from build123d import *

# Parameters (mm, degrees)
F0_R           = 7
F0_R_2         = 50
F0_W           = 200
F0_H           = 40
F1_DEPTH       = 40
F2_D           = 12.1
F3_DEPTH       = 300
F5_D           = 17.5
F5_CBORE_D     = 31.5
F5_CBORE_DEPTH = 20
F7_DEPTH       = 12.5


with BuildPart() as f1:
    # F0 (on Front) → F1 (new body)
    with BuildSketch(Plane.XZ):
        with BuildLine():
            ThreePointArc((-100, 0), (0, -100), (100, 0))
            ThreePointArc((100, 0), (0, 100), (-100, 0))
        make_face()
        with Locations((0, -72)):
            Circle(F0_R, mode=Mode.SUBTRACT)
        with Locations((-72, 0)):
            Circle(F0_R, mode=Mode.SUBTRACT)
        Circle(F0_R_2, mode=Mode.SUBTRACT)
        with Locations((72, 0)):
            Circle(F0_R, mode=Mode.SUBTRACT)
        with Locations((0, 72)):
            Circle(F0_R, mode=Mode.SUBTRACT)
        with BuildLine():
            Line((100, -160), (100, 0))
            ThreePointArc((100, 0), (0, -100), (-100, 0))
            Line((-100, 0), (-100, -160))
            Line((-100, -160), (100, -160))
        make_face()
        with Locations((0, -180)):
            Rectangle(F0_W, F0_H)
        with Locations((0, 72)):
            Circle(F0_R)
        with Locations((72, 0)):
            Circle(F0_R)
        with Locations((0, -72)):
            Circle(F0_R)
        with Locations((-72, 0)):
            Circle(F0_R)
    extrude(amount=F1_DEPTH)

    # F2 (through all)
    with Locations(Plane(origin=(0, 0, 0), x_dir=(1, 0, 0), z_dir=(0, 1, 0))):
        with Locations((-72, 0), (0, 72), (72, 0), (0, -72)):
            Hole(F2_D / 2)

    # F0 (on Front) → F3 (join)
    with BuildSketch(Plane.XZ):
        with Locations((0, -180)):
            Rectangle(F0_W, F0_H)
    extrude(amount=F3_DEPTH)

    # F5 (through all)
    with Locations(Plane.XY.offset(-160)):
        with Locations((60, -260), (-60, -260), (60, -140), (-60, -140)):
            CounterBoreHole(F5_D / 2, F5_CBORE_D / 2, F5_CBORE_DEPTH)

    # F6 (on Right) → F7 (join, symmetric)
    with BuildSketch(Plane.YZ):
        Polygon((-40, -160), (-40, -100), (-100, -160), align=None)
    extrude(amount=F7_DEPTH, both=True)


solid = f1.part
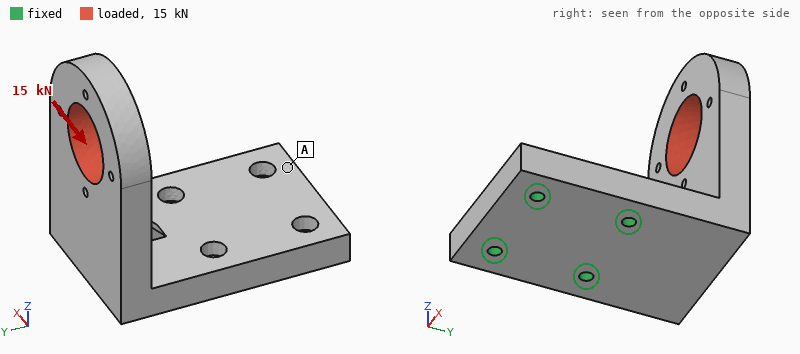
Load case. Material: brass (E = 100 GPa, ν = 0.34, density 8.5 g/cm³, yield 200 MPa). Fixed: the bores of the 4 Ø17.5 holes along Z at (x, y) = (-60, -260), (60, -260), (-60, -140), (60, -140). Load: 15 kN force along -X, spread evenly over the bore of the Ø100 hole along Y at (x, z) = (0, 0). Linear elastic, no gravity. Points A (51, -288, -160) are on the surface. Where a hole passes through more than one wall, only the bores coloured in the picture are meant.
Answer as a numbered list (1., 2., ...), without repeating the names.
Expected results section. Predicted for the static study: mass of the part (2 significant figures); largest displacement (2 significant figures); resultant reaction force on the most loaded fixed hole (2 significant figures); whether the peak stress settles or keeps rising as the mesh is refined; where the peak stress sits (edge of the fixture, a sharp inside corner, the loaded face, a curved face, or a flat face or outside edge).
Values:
1. 33 kg
2. 0.41 mm
3. 29 kN
4. keeps rising
5. edge of the fixture
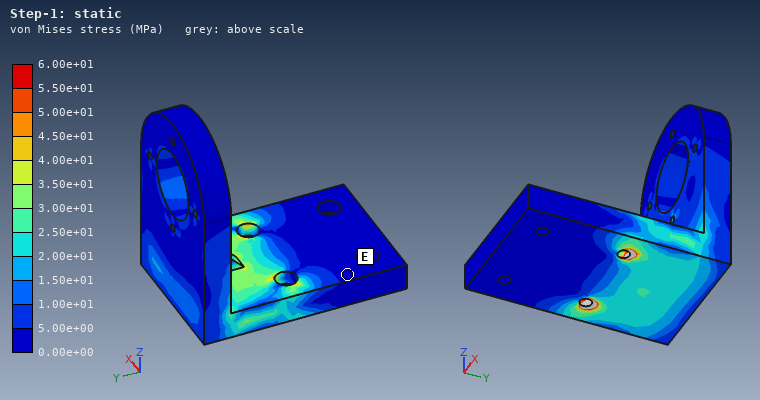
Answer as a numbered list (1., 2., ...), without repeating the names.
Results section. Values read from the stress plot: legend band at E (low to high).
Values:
1. 0.00e+00 to 5.00e+00 MPa
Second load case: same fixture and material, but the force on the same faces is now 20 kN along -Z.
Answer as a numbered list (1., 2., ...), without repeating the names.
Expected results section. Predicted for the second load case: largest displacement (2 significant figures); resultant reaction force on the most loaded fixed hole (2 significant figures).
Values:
1. 0.56 mm
2. 21 kN
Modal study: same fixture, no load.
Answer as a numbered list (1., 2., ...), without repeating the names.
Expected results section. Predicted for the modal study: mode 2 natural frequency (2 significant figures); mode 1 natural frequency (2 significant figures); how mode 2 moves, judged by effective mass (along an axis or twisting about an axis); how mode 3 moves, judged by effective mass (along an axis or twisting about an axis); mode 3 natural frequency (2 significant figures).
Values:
1. 360 Hz
2. 210 Hz
3. along X
4. along Z
5. 640 Hz
